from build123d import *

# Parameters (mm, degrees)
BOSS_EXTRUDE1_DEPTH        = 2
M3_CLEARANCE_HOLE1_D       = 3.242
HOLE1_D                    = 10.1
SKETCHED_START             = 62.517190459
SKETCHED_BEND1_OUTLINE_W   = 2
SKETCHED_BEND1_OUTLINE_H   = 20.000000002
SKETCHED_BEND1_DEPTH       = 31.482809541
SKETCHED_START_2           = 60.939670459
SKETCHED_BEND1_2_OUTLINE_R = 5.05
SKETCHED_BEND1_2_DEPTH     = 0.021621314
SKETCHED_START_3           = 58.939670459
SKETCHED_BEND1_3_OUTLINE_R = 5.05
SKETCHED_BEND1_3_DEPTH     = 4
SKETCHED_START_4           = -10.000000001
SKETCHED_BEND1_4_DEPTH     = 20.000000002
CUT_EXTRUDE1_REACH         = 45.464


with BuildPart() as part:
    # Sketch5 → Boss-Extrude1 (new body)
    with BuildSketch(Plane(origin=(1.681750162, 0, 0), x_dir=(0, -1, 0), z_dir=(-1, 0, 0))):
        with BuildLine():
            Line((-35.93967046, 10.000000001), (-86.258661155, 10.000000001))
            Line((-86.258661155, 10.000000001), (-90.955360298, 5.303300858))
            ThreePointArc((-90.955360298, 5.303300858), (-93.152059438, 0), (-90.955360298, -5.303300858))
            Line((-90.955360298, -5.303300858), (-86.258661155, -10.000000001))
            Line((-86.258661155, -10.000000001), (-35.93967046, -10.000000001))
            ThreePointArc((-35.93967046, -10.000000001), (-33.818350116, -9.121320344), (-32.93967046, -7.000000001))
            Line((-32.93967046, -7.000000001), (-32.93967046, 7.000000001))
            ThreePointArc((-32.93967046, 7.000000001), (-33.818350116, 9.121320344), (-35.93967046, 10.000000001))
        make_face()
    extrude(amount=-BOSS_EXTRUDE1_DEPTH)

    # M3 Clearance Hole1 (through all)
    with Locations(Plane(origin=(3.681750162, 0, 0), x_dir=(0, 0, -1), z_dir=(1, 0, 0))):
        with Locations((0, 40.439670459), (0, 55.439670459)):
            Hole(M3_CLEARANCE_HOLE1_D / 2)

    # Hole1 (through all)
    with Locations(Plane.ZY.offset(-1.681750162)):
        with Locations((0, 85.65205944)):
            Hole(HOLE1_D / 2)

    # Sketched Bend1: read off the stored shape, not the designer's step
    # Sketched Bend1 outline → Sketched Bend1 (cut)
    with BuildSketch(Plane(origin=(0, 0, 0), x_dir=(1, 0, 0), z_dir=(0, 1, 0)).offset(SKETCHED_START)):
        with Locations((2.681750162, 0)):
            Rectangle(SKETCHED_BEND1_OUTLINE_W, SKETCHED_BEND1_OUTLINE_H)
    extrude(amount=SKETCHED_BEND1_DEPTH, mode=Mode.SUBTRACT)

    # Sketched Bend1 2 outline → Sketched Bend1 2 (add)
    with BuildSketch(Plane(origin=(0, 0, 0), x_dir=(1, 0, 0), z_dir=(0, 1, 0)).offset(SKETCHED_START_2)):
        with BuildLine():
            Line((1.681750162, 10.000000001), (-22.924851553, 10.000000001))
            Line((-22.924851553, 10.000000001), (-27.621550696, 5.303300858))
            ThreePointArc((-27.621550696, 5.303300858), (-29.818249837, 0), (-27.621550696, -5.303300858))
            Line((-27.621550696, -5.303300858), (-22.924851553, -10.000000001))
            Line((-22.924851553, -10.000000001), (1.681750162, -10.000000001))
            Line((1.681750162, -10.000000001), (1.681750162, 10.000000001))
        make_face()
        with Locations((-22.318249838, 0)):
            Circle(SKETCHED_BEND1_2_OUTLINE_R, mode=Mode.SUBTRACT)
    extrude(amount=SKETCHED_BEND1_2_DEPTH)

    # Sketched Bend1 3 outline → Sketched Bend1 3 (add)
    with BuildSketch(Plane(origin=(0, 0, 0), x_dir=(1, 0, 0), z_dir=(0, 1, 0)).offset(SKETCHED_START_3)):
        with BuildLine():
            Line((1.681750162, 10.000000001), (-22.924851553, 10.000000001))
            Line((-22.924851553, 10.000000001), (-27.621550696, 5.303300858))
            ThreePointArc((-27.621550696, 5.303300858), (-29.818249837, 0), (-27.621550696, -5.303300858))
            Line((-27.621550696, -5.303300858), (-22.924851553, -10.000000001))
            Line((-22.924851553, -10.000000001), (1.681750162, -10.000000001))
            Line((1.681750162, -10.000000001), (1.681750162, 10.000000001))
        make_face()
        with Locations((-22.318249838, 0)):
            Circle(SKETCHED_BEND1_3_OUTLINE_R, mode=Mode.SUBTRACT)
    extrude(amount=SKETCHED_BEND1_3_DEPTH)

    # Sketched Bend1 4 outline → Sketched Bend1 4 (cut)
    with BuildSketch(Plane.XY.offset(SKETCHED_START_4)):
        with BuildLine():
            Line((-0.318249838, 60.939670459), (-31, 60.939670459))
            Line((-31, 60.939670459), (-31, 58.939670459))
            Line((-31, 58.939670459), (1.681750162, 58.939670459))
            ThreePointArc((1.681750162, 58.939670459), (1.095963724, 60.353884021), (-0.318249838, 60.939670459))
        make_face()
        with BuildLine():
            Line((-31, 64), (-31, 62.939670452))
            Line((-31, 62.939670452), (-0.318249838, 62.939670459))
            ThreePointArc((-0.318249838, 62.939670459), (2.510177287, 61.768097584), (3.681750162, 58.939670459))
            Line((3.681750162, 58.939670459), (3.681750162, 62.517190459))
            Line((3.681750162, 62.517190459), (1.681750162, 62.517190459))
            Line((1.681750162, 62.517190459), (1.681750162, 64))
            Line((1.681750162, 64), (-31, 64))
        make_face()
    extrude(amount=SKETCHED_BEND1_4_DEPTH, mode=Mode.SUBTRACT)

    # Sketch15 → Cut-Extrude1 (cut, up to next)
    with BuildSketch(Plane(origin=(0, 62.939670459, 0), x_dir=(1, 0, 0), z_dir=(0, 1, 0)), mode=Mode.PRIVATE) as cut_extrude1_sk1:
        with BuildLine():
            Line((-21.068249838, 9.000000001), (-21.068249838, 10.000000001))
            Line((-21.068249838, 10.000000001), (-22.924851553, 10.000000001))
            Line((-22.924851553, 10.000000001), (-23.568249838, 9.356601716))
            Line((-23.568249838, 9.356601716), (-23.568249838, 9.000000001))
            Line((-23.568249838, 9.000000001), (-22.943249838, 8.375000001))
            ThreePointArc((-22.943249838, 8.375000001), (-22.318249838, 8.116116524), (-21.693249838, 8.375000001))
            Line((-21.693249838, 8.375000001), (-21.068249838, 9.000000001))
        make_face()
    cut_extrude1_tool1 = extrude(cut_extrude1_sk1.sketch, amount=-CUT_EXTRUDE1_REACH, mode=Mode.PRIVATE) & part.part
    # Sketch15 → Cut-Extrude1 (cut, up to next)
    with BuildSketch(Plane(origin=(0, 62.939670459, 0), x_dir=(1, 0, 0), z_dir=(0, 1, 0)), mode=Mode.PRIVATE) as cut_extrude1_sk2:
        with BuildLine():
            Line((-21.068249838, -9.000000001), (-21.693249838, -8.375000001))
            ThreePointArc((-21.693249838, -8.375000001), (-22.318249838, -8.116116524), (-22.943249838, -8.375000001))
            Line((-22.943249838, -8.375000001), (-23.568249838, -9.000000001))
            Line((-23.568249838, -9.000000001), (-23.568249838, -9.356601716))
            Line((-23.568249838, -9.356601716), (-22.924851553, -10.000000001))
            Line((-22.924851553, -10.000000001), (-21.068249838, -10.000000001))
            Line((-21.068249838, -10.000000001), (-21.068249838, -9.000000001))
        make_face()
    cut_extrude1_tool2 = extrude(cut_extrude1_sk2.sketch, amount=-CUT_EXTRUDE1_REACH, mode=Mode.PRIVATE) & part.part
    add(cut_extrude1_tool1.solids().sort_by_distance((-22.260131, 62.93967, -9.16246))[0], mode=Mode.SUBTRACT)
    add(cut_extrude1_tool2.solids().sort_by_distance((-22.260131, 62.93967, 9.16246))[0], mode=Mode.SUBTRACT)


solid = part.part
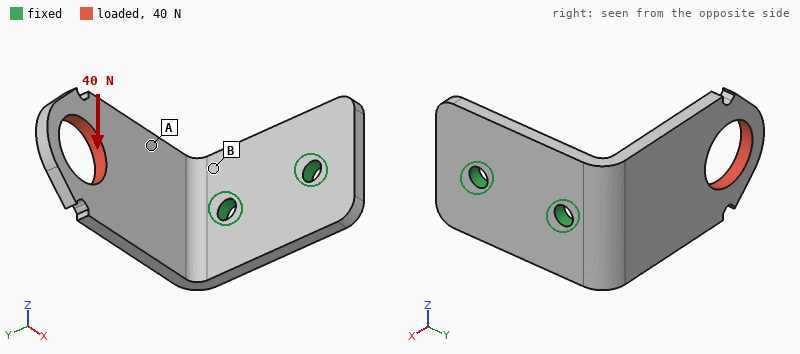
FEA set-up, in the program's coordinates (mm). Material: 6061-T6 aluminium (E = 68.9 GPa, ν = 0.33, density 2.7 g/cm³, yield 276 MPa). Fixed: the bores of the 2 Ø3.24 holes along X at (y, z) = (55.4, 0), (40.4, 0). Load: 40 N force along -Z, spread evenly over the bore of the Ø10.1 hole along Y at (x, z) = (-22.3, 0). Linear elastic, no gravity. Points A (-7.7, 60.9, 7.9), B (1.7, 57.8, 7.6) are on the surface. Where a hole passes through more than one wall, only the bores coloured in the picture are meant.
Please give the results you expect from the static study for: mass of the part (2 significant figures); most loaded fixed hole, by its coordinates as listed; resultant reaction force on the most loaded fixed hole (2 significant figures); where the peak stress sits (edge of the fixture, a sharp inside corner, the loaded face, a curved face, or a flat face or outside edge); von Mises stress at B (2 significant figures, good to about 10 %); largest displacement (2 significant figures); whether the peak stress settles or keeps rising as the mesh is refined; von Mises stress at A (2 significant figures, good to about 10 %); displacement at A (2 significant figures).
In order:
5.7 g
(55.4, 0)
50 N
edge of the fixture
22 MPa
0.12 mm
keeps rising
9.4 MPa
0.048 mm
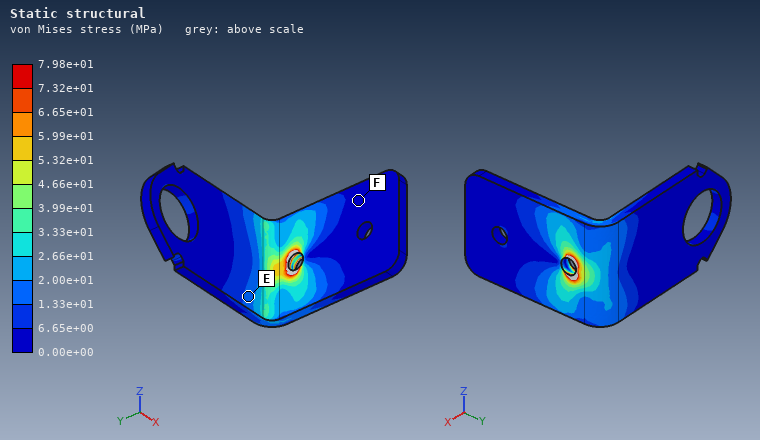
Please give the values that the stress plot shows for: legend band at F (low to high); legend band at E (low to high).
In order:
0.00e+00 to 6.65e+00 MPa
1.33e+01 to 2.00e+01 MPa
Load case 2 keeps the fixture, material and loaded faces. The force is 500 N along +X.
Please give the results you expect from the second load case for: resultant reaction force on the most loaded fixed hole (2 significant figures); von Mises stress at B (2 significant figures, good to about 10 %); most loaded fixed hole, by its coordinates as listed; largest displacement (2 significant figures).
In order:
550 N
85 MPa
(55.4, 0)
0.38 mm
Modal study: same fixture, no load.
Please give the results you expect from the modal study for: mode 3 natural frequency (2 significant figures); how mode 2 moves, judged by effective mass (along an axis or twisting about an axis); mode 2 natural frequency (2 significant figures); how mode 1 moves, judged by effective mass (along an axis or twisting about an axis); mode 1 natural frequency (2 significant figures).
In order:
6300 Hz
along Z
3000 Hz
along Y
1700 Hz
